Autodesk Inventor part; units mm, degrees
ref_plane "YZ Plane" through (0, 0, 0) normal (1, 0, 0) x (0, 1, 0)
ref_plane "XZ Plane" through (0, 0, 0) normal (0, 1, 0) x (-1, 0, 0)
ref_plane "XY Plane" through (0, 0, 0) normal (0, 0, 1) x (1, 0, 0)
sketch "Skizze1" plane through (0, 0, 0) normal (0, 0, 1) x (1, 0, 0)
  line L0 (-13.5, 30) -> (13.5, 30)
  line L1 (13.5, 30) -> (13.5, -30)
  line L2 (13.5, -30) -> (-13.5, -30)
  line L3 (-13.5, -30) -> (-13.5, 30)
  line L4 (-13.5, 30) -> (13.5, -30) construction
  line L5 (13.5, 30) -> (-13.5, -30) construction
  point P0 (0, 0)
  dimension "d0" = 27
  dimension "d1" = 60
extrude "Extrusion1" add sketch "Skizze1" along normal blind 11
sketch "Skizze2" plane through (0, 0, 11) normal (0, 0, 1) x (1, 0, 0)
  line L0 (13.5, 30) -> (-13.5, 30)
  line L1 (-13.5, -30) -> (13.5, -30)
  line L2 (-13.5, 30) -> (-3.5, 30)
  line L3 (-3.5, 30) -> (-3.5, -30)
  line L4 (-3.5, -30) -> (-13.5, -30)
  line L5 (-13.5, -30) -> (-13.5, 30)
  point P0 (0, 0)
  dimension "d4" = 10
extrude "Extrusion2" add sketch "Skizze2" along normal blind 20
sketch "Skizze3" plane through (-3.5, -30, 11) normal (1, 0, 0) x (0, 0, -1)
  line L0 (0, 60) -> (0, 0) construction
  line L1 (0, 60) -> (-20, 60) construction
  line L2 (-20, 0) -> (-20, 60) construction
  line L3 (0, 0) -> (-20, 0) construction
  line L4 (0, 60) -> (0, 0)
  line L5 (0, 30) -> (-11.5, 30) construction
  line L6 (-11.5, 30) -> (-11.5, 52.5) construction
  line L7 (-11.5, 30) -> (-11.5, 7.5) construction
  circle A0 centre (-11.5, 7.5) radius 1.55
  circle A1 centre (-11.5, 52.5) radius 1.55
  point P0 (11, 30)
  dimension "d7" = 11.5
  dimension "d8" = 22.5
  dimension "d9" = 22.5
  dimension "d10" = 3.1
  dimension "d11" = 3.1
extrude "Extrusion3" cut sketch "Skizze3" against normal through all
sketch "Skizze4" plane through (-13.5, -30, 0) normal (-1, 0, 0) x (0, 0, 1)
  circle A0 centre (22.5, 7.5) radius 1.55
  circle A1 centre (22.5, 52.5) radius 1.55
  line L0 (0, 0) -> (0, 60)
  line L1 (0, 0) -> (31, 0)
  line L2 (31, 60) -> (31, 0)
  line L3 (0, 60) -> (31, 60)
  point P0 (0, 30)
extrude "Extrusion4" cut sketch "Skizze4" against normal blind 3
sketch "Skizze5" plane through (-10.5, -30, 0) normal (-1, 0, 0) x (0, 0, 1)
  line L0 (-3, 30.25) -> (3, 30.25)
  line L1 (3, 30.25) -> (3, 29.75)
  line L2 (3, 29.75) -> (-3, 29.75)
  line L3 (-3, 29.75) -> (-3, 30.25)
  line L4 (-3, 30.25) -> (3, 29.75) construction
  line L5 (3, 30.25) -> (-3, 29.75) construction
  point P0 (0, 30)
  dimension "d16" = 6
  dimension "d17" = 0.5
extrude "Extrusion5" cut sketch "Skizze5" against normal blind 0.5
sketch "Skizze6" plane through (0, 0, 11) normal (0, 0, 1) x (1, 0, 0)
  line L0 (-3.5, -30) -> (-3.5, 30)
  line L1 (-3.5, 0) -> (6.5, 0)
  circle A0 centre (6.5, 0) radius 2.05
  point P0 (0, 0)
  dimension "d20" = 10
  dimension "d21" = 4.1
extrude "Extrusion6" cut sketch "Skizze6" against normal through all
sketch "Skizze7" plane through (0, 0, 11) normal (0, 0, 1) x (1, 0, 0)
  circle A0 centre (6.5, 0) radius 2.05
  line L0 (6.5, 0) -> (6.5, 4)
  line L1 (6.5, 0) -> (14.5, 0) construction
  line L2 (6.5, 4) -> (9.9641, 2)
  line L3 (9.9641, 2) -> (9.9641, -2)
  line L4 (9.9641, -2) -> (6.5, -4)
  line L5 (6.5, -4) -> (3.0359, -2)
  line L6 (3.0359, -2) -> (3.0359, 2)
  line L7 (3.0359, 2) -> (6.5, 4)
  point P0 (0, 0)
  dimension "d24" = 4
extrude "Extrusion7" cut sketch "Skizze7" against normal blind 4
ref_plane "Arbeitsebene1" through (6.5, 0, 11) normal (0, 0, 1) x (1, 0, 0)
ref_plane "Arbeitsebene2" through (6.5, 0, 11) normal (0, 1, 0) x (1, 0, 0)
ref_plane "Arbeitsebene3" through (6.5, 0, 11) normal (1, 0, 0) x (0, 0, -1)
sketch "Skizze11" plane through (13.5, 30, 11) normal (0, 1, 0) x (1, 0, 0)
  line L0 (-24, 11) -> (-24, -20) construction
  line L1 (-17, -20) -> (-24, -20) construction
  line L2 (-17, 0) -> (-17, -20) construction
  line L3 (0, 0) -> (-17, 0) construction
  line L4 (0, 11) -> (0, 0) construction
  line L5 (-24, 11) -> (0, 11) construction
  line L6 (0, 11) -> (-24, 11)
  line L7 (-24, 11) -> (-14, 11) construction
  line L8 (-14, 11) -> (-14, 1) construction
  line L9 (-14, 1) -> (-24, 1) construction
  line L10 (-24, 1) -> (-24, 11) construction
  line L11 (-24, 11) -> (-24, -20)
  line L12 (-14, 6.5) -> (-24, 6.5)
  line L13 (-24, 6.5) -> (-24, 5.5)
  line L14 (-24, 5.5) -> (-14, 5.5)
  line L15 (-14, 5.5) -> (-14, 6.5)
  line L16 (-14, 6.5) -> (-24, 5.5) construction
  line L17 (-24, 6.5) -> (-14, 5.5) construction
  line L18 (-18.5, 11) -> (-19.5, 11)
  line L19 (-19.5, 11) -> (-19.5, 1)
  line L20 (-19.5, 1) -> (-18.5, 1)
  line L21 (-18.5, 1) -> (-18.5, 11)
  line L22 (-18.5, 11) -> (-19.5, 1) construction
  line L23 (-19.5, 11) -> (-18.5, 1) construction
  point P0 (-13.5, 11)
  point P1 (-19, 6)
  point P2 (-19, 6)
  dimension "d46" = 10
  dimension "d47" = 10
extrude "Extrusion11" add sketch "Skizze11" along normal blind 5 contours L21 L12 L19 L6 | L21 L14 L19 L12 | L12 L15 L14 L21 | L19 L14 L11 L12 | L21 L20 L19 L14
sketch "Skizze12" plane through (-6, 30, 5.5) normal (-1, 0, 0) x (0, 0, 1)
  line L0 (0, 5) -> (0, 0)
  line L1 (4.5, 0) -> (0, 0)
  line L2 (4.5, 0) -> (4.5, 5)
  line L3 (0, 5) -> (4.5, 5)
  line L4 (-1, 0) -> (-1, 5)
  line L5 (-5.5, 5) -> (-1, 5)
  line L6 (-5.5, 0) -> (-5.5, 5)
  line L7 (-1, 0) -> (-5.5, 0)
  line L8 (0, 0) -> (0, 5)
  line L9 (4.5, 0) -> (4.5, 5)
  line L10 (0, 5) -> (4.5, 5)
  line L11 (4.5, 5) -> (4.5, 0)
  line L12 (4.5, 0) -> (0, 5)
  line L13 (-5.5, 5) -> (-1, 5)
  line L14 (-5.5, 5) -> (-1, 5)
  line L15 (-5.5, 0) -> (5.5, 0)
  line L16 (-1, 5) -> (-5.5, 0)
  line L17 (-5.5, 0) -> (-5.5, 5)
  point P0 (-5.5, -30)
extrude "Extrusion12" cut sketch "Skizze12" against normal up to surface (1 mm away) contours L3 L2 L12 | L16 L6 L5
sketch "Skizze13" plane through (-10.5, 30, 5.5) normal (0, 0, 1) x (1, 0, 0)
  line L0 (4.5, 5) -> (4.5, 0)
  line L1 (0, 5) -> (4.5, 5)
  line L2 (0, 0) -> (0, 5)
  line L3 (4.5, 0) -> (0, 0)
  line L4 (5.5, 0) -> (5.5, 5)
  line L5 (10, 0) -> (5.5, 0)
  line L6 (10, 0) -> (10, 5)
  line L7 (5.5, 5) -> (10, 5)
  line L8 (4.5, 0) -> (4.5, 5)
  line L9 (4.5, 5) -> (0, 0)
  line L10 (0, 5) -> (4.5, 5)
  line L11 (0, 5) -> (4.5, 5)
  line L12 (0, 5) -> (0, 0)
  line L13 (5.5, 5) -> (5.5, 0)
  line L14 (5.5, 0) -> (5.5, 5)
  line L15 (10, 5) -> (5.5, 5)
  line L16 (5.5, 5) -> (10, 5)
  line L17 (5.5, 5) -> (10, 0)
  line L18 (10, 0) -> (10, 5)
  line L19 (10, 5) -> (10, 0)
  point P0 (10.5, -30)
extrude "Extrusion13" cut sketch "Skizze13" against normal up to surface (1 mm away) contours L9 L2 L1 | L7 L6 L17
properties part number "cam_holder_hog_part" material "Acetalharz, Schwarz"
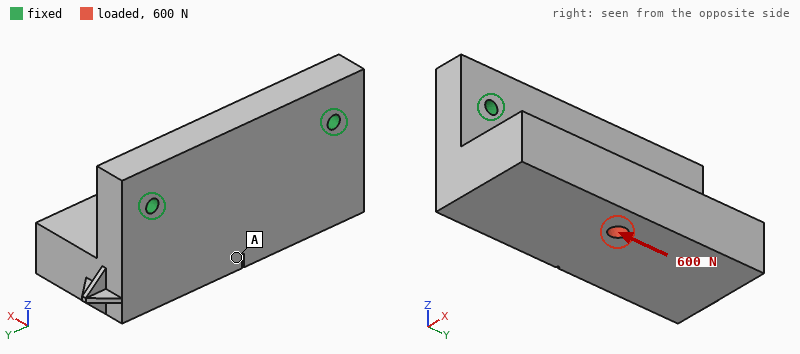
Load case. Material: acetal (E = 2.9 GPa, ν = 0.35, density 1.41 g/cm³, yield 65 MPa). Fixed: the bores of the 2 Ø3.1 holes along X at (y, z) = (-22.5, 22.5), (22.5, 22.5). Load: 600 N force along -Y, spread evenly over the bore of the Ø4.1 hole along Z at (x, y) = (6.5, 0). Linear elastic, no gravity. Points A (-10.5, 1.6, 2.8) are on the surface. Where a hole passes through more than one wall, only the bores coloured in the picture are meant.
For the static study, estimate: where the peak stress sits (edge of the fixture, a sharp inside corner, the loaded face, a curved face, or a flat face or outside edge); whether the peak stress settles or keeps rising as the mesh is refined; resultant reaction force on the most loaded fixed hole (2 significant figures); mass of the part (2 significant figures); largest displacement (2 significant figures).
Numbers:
edge of the fixture
keeps rising
420 N
34 g
0.16 mm
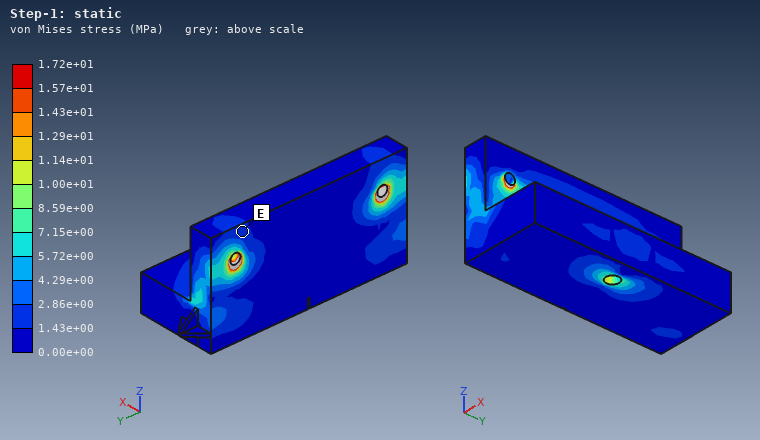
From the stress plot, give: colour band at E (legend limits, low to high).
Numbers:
1.43e+00 to 2.86e+00 MPa
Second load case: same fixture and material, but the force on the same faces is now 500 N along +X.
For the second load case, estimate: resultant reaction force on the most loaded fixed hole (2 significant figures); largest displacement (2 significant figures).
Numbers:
250 N
0.83 mm
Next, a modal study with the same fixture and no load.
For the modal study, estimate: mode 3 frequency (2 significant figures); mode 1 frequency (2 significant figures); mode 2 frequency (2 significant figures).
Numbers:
3300 Hz
990 Hz
2200 Hz
